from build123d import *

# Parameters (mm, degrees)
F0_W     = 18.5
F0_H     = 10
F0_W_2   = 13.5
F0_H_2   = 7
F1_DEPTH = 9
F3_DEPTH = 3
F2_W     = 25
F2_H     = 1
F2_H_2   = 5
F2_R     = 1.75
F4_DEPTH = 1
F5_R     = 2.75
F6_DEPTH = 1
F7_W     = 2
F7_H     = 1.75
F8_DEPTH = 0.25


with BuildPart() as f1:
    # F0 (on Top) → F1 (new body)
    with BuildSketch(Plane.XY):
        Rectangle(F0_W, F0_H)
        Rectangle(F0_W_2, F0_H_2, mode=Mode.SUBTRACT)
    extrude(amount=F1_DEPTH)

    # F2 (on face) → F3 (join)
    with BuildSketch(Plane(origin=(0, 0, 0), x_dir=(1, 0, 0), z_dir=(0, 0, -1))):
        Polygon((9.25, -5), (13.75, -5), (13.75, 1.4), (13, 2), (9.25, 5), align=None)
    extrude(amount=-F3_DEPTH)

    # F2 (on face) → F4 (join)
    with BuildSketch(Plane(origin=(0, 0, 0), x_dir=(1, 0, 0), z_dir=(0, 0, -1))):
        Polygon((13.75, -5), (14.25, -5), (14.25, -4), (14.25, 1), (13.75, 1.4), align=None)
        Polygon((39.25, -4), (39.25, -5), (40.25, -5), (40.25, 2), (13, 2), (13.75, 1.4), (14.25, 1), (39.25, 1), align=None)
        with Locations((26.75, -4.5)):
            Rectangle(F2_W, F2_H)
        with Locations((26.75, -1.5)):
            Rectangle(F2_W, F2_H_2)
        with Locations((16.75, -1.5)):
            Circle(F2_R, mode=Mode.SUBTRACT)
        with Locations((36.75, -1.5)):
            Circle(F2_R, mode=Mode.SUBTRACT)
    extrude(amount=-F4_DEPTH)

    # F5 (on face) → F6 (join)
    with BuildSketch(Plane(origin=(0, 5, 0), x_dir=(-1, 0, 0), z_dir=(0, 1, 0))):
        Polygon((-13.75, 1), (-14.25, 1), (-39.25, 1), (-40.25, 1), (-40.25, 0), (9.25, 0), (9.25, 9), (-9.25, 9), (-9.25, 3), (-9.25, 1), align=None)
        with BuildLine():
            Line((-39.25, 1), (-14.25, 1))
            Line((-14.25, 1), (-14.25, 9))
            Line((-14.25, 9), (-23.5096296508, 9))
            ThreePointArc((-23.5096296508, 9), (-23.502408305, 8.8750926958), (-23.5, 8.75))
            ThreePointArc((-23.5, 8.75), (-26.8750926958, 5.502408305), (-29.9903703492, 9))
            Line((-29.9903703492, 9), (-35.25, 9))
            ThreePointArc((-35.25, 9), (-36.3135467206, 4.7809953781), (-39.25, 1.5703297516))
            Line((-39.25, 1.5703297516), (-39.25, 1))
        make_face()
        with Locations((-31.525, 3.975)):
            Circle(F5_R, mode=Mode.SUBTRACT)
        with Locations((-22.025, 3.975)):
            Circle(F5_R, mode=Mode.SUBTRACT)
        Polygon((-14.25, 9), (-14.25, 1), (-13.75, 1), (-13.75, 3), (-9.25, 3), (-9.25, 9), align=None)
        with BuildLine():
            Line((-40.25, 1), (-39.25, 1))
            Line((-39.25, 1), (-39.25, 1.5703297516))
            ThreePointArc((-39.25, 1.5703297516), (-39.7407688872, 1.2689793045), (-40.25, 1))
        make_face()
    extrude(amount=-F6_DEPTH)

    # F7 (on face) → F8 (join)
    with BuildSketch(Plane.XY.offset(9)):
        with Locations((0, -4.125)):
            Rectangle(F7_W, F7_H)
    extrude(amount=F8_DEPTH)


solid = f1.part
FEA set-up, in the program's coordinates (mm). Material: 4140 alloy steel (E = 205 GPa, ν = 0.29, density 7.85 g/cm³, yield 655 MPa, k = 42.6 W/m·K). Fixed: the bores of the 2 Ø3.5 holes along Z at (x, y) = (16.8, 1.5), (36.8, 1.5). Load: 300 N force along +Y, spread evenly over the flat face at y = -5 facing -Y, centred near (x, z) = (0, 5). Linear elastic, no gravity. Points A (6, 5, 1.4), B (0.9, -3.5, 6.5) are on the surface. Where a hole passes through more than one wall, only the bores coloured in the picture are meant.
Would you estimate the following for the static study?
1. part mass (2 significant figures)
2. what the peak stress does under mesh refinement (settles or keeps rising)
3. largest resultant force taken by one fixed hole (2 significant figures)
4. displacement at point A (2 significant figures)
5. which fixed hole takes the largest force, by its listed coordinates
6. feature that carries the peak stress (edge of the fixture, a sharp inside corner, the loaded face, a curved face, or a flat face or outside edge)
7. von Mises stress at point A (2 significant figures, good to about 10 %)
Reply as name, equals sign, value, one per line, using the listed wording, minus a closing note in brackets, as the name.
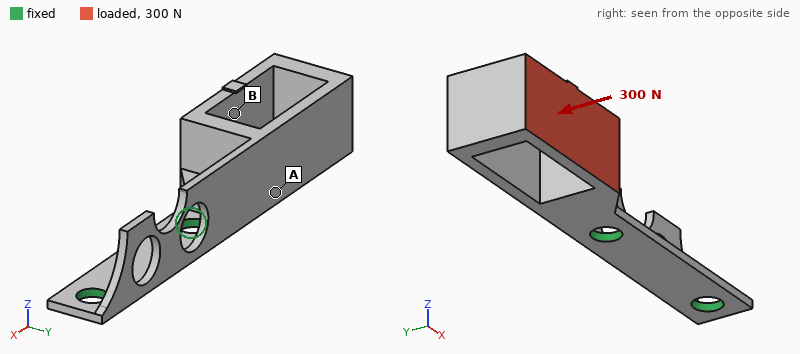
part mass = 9.7 g
what the peak stress does under mesh refinement = keeps rising
largest resultant force taken by one fixed hole = 350 N
displacement at point A = 0.045 mm
which fixed hole takes the largest force, by its listed coordinates = (16.8, 1.5)
feature that carries the peak stress = edge of the fixture
von Mises stress at point A = 160 MPa
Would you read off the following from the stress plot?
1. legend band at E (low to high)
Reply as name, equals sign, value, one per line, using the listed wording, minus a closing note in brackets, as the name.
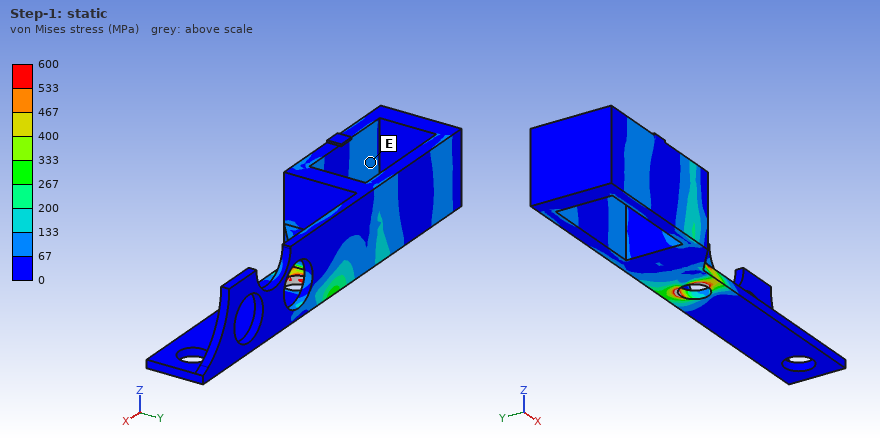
legend band at E = 67 to 133 MPa
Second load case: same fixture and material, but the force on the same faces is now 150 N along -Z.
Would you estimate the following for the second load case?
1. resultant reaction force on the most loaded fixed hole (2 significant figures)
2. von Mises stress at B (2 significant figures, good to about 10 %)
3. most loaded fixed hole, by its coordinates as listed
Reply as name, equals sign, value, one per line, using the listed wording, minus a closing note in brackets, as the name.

resultant reaction force on the most loaded fixed hole = 240 N
von Mises stress at B = 29 MPa
most loaded fixed hole, by its coordinates as listed = (16.8, 1.5)
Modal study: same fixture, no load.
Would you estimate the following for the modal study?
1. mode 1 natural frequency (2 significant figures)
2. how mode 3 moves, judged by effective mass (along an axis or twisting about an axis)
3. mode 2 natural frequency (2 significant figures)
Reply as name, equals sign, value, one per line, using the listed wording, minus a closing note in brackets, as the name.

mode 1 natural frequency = 2700 Hz
how mode 3 moves, judged by effective mass = twisting about X
mode 2 natural frequency = 3600 Hz
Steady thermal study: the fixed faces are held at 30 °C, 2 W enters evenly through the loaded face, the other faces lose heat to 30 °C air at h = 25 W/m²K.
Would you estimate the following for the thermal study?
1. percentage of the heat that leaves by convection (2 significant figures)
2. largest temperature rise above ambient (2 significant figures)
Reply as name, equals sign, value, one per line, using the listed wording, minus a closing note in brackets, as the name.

percentage of the heat that leaves by convection = 28 %
largest temperature rise above ambient = 30 K
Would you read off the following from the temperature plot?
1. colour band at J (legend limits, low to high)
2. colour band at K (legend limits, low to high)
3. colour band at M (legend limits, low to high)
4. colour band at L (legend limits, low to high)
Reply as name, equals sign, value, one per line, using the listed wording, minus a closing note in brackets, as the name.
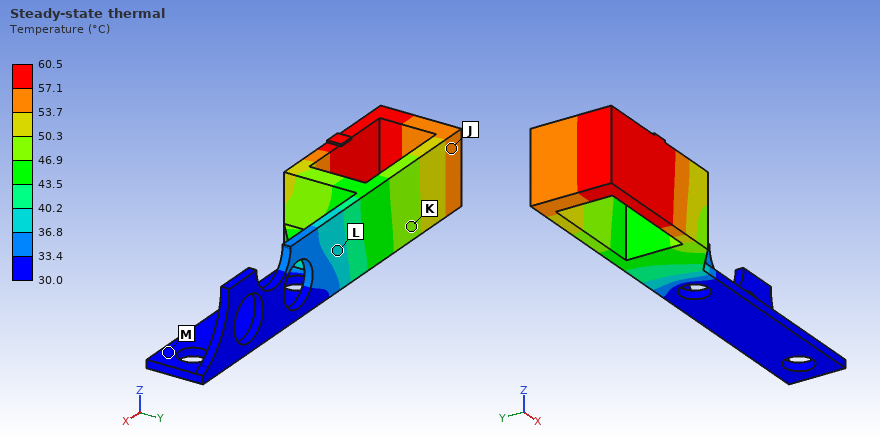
colour band at J = 53.7 to 57.1 °C
colour band at K = 46.9 to 50.3 °C
colour band at M = 30.0 to 33.4 °C
colour band at L = 36.8 to 40.2 °C
